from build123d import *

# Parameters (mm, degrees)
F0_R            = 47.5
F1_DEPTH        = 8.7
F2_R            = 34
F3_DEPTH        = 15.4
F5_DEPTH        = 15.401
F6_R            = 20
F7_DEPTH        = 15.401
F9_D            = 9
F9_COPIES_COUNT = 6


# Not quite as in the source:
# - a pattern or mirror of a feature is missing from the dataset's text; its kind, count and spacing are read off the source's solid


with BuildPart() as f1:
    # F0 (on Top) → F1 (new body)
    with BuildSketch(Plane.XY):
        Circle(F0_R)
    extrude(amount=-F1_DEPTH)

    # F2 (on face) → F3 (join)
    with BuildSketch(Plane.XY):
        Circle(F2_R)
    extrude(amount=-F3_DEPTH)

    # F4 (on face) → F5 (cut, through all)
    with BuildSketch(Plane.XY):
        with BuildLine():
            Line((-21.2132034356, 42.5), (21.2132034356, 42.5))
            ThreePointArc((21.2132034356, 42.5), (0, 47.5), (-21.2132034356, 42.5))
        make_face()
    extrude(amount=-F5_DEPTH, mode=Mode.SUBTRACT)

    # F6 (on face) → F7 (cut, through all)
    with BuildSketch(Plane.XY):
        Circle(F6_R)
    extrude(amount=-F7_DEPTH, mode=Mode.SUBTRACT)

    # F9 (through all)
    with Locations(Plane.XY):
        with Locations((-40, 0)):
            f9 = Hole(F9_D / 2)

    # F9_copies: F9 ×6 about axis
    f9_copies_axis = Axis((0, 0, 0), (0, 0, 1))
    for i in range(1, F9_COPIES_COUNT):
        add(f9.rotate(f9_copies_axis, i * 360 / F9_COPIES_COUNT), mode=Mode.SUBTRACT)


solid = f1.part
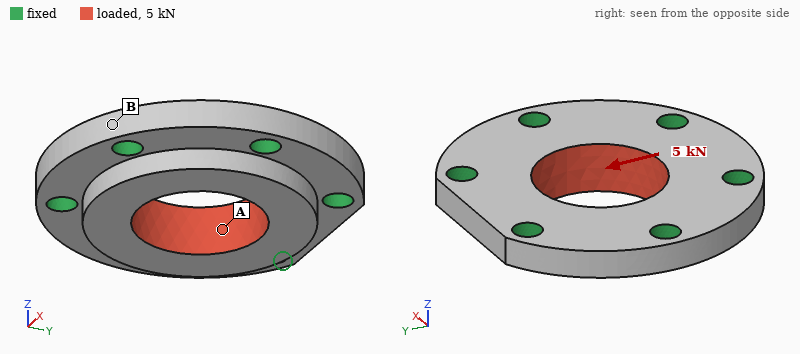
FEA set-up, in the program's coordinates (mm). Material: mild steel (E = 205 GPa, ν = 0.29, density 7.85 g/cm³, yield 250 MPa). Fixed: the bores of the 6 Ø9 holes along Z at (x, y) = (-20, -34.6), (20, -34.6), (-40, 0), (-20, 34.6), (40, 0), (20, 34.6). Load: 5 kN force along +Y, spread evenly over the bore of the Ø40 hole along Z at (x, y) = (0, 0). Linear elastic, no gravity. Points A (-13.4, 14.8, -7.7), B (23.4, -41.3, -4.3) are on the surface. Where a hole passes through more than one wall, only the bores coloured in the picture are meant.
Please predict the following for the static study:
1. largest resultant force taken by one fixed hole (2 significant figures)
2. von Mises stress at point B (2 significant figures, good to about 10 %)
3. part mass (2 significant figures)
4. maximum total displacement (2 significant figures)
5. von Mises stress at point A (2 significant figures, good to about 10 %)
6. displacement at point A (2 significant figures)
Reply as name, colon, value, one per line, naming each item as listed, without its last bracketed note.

largest resultant force taken by one fixed hole: 1.0 kN
von Mises stress at point B: 1.8 MPa
part mass: 490 g
maximum total displacement: 0.85 µm
von Mises stress at point A: 4.5 MPa
displacement at point A: 0.53 µm
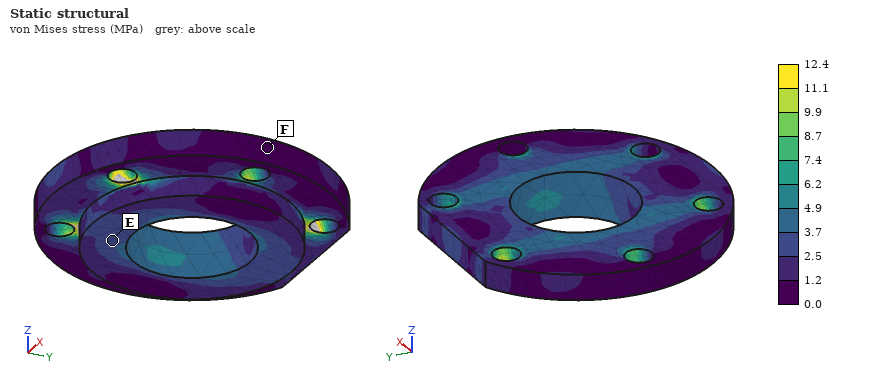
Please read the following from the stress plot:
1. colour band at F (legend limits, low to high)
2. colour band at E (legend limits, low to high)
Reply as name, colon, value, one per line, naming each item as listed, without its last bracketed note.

colour band at F: 0.0 to 1.2 MPa
colour band at E: 2.5 to 3.7 MPa
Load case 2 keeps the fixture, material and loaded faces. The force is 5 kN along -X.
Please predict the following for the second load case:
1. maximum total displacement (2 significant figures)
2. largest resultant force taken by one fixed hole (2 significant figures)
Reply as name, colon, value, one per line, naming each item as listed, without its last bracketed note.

maximum total displacement: 0.77 µm
largest resultant force taken by one fixed hole: 1.1 kN
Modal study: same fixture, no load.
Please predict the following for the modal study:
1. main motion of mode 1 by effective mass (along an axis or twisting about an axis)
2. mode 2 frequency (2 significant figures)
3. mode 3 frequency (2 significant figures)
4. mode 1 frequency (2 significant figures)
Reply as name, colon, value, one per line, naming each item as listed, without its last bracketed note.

main motion of mode 1 by effective mass: along Z
mode 2 frequency: 23 kHz
mode 3 frequency: 23 kHz
mode 1 frequency: 18 kHz
